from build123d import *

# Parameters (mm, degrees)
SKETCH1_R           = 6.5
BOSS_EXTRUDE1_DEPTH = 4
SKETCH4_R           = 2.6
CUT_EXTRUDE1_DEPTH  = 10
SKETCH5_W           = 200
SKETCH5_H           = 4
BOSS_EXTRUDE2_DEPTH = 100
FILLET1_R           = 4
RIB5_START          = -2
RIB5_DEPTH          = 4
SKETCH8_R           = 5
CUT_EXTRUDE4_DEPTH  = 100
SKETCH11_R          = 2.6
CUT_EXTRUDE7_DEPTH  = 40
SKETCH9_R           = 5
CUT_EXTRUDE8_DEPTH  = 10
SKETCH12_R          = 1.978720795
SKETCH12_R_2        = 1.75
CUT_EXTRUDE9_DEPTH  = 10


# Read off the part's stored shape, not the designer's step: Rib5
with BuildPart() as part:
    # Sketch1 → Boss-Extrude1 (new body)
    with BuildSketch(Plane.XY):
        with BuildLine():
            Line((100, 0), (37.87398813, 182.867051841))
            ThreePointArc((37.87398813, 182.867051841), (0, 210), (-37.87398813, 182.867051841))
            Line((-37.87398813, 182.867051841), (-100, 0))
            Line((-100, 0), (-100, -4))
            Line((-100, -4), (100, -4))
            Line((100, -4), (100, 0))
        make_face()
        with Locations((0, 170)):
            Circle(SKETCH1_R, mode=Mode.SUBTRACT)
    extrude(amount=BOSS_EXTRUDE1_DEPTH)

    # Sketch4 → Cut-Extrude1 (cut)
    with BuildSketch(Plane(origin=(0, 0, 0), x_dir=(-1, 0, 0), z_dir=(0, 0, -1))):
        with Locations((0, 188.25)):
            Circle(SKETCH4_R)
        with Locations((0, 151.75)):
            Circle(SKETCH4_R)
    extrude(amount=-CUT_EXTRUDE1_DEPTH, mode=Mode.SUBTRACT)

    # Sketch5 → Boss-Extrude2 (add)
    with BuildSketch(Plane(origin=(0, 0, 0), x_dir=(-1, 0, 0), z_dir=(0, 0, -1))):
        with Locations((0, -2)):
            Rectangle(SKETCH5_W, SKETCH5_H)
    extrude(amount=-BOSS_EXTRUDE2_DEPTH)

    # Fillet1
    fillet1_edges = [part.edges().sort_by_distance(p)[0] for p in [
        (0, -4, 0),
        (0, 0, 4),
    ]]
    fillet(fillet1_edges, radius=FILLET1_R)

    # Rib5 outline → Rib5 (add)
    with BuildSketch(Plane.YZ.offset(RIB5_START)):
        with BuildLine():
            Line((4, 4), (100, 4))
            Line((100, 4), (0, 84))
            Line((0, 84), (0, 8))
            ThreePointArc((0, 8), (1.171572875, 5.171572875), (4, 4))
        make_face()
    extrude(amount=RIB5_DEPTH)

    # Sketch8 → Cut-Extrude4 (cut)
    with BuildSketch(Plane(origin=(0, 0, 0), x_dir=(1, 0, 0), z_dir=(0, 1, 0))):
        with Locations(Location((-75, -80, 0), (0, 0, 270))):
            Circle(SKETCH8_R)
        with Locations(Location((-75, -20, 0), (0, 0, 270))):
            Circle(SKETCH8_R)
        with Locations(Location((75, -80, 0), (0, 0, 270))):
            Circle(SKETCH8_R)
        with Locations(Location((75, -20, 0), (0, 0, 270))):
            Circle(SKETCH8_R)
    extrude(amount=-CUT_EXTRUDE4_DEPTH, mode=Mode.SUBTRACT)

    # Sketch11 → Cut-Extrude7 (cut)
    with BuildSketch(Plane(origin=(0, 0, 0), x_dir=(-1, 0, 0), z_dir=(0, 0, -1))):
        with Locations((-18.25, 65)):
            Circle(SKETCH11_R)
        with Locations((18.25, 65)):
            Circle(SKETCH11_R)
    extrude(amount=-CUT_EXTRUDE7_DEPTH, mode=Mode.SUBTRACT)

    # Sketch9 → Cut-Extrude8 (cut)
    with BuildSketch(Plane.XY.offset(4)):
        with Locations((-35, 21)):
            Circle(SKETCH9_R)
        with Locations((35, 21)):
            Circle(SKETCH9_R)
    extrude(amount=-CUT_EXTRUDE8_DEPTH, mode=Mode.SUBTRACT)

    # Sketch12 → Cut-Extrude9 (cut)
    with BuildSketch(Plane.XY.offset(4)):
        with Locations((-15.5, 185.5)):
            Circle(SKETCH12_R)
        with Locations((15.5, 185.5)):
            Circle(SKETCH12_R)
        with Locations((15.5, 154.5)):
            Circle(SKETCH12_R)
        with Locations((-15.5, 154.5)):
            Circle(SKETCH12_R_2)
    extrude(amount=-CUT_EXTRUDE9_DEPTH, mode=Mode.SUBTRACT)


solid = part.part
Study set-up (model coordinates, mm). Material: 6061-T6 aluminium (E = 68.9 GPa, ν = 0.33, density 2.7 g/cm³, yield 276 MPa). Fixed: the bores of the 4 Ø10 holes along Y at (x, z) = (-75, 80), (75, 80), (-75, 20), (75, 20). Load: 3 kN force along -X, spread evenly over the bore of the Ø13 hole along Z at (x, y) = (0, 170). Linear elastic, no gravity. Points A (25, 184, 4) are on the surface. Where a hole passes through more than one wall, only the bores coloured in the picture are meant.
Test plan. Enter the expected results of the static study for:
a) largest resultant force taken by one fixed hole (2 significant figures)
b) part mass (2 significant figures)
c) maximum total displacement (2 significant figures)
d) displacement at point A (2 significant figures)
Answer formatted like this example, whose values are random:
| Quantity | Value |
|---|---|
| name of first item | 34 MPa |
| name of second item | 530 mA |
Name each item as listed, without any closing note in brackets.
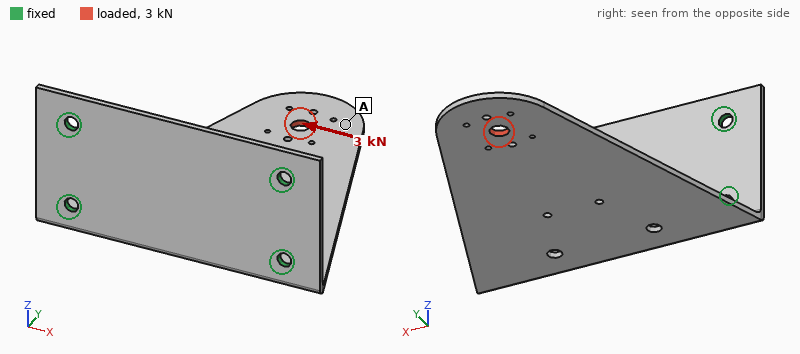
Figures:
| Quantity | Value |
|---|---|
| largest resultant force taken by one fixed hole | 3.8 kN |
| part mass | 540 g |
| maximum total displacement | 0.73 mm |
| displacement at point A | 0.68 mm |
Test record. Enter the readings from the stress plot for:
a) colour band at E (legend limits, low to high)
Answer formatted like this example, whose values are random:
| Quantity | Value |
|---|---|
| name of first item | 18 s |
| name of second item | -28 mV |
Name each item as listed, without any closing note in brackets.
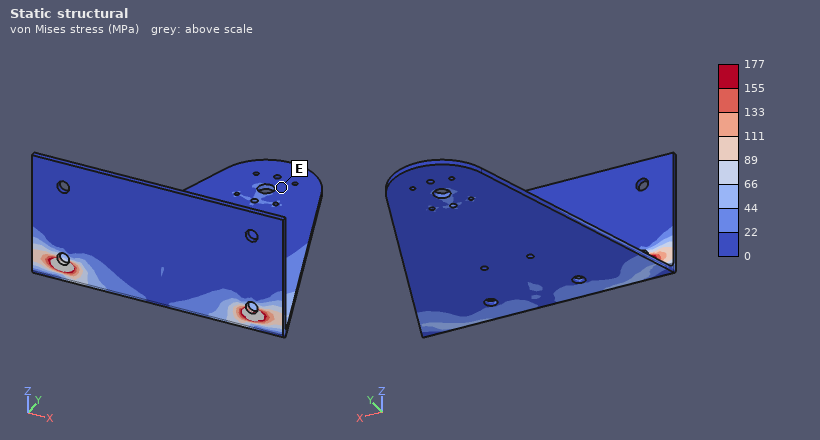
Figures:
| Quantity | Value |
|---|---|
| colour band at E | 0 to 22 MPa |
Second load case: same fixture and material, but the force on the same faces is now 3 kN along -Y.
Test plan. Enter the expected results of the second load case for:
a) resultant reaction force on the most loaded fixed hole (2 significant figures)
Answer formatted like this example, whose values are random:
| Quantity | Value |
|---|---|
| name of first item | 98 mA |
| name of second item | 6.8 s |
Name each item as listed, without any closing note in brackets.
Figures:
| Quantity | Value |
|---|---|
| resultant reaction force on the most loaded fixed hole | 1.7 kN |
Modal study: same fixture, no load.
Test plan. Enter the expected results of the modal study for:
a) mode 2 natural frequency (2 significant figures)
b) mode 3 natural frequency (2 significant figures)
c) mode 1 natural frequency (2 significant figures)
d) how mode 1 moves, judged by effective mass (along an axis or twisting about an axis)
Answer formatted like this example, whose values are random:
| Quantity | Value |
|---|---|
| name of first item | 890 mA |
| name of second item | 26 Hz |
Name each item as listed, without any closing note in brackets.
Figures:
| Quantity | Value |
|---|---|
| mode 2 natural frequency | 430 Hz |
| mode 3 natural frequency | 550 Hz |
| mode 1 natural frequency | 200 Hz |
| how mode 1 moves, judged by effective mass | along Z |
